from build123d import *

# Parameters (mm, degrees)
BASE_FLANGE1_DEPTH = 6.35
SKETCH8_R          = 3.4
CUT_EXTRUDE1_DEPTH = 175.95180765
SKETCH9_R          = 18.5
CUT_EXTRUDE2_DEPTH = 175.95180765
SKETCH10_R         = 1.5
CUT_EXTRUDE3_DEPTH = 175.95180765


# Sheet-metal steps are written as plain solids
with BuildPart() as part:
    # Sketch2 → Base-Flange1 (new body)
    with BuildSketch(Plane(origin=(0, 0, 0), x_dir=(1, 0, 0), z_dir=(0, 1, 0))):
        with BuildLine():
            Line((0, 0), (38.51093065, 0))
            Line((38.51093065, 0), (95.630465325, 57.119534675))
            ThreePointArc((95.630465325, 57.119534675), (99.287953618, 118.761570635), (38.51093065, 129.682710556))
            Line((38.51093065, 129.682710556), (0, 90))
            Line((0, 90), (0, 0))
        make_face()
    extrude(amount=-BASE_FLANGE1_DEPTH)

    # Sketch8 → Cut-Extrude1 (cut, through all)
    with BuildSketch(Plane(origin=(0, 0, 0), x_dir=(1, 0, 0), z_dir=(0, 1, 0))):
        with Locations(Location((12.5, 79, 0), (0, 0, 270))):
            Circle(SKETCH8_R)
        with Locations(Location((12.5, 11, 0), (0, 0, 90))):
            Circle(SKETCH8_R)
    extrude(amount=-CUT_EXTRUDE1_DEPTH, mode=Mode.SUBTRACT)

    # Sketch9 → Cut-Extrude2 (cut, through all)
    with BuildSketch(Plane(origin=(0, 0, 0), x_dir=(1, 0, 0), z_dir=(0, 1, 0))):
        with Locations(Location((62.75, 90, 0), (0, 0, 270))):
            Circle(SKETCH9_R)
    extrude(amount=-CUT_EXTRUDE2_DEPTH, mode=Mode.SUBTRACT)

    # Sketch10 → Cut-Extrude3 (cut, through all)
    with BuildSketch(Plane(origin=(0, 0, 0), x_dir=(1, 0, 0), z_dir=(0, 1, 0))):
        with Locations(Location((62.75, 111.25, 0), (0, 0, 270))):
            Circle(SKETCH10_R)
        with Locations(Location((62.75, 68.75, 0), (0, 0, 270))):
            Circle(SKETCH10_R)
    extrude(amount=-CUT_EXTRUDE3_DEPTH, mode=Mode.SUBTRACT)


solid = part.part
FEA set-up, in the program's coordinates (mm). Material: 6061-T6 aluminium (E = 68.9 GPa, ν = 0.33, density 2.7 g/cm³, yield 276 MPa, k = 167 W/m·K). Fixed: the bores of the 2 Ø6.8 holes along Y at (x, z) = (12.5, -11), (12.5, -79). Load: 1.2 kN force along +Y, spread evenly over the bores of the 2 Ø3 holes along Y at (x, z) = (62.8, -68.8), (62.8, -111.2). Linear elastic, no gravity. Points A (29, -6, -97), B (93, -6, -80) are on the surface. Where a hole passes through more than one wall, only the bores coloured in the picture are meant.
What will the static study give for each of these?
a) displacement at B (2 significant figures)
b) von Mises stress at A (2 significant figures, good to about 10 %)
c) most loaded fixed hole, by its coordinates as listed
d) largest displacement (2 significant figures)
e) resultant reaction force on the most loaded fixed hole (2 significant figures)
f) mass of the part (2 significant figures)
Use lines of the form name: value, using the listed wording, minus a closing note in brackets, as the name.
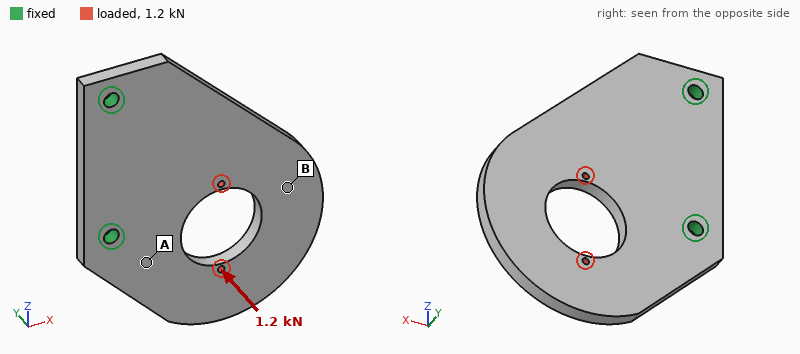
displacement at B: 0.95 mm
von Mises stress at A: 68 MPa
most loaded fixed hole, by its coordinates as listed: (12.5, -79)
largest displacement: 1.3 mm
resultant reaction force on the most loaded fixed hole: 1.3 kN
mass of the part: 170 g
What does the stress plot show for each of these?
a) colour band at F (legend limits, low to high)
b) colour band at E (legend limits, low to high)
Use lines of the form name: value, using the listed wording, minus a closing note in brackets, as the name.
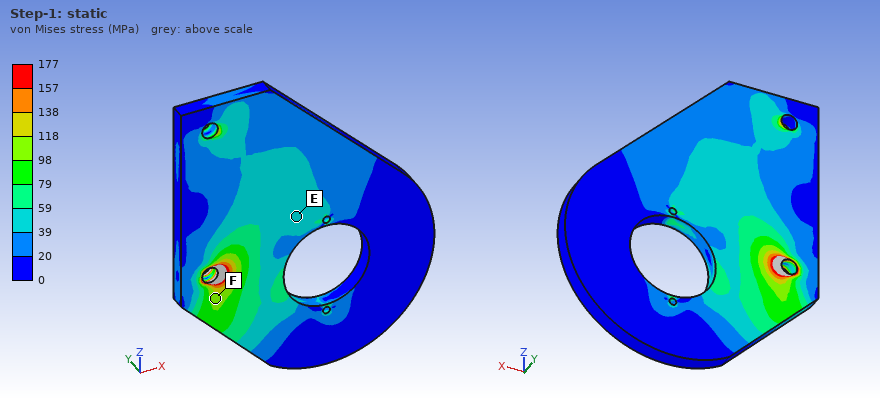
colour band at F: 98 to 118 MPa
colour band at E: 39 to 59 MPa
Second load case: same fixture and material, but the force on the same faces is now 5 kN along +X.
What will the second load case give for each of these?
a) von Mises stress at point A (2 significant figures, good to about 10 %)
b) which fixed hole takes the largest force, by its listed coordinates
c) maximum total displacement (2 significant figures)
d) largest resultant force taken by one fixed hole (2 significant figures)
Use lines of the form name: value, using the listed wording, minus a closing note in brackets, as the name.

von Mises stress at point A: 21 MPa
which fixed hole takes the largest force, by its listed coordinates: (12.5, -79)
maximum total displacement: 60 µm
largest resultant force taken by one fixed hole: 5.6 kN
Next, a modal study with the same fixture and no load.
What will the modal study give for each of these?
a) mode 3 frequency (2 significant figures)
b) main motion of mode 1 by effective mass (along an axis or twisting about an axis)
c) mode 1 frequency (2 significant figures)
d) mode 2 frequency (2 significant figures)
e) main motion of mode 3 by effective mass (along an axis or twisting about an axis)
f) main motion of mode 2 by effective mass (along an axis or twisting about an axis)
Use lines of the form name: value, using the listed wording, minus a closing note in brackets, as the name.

mode 3 frequency: 2500 Hz
main motion of mode 1 by effective mass: along Y
mode 1 frequency: 570 Hz
mode 2 frequency: 1300 Hz
main motion of mode 3 by effective mass: along Y
main motion of mode 2 by effective mass: twisting about X
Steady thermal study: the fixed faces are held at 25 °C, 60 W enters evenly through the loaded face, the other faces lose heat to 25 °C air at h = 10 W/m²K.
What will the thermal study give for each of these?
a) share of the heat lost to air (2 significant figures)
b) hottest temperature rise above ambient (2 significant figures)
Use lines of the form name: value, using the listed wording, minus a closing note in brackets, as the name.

share of the heat lost to air: 9.4 %
hottest temperature rise above ambient: 62 K
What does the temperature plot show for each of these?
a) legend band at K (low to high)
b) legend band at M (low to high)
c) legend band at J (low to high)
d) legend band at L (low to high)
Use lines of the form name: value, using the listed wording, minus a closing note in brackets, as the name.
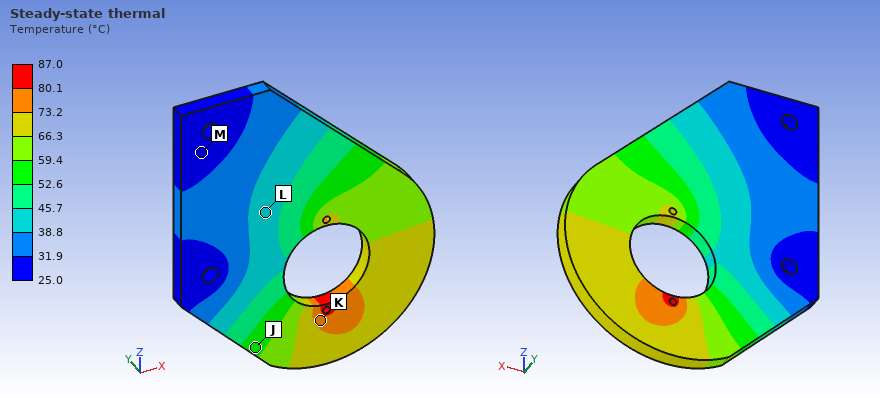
legend band at K: 73.2 to 80.1 °C
legend band at M: 25.0 to 31.9 °C
legend band at J: 52.6 to 59.4 °C
legend band at L: 38.8 to 45.7 °C
